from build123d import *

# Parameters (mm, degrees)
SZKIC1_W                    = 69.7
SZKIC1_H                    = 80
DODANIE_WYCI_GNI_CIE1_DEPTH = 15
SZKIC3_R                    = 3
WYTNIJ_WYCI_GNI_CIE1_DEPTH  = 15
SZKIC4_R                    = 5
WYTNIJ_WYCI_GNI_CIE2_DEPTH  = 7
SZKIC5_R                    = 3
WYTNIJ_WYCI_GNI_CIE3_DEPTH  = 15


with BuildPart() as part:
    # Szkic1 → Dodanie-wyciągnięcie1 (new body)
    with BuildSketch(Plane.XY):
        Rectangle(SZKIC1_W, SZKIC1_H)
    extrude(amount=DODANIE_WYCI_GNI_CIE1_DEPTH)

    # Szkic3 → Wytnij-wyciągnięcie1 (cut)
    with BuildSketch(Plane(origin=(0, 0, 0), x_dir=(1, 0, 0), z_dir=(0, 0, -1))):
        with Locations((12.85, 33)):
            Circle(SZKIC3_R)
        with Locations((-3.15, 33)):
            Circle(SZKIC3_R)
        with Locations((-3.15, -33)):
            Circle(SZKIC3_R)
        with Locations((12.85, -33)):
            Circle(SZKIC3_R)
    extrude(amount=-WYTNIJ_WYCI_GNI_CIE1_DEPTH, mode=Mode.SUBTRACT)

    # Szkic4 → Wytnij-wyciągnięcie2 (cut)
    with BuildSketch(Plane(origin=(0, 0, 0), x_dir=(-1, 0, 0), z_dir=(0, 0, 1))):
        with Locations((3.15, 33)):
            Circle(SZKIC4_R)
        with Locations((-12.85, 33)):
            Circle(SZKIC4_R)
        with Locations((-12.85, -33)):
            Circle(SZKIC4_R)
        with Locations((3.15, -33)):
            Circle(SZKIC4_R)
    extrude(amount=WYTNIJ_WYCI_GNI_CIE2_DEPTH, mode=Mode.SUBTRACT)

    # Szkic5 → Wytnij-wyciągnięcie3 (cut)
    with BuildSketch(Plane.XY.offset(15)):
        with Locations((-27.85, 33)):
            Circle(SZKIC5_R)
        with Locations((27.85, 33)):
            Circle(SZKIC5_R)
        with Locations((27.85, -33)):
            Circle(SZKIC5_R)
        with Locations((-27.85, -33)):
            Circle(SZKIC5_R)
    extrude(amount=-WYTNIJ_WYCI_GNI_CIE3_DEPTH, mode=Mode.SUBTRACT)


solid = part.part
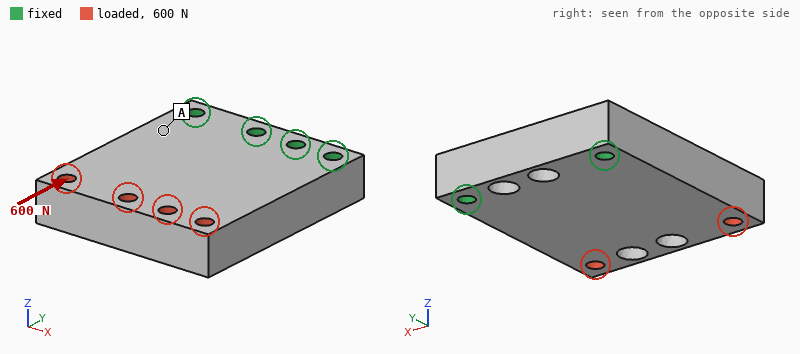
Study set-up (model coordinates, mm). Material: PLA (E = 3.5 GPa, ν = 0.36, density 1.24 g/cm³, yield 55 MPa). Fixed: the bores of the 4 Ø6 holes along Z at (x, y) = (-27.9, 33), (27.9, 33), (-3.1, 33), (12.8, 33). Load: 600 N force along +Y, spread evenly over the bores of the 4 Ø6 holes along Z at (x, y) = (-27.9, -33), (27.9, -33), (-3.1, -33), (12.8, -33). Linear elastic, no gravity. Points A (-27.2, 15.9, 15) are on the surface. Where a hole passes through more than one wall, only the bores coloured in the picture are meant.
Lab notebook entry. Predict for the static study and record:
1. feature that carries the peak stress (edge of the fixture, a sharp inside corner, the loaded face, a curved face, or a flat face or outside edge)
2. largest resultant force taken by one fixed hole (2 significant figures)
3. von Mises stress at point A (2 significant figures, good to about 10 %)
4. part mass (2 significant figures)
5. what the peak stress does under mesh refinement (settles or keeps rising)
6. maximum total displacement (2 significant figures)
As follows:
edge of the fixture
180 N
0.79 MPa
98 g
keeps rising
28 µm
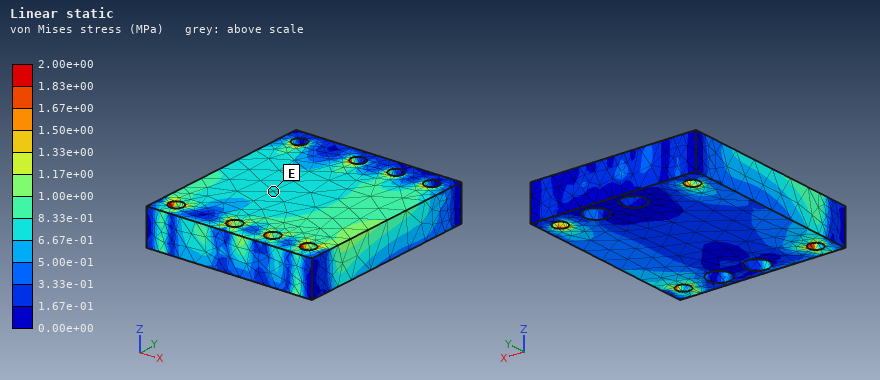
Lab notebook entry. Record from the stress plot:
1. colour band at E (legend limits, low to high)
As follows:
6.67e-01 to 8.33e-01 MPa
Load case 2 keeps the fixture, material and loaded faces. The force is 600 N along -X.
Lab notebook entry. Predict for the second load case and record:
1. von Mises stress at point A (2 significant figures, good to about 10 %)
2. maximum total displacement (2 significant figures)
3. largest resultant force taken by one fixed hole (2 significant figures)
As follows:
2.1 MPa
97 µm
710 N
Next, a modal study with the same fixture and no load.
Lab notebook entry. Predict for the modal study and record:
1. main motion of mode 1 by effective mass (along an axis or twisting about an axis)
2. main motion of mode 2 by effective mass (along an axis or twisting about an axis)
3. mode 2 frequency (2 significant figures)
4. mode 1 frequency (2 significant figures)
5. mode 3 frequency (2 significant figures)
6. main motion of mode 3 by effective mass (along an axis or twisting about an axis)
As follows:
along Z
twisting about Y
1700 Hz
720 Hz
2400 Hz
along X
